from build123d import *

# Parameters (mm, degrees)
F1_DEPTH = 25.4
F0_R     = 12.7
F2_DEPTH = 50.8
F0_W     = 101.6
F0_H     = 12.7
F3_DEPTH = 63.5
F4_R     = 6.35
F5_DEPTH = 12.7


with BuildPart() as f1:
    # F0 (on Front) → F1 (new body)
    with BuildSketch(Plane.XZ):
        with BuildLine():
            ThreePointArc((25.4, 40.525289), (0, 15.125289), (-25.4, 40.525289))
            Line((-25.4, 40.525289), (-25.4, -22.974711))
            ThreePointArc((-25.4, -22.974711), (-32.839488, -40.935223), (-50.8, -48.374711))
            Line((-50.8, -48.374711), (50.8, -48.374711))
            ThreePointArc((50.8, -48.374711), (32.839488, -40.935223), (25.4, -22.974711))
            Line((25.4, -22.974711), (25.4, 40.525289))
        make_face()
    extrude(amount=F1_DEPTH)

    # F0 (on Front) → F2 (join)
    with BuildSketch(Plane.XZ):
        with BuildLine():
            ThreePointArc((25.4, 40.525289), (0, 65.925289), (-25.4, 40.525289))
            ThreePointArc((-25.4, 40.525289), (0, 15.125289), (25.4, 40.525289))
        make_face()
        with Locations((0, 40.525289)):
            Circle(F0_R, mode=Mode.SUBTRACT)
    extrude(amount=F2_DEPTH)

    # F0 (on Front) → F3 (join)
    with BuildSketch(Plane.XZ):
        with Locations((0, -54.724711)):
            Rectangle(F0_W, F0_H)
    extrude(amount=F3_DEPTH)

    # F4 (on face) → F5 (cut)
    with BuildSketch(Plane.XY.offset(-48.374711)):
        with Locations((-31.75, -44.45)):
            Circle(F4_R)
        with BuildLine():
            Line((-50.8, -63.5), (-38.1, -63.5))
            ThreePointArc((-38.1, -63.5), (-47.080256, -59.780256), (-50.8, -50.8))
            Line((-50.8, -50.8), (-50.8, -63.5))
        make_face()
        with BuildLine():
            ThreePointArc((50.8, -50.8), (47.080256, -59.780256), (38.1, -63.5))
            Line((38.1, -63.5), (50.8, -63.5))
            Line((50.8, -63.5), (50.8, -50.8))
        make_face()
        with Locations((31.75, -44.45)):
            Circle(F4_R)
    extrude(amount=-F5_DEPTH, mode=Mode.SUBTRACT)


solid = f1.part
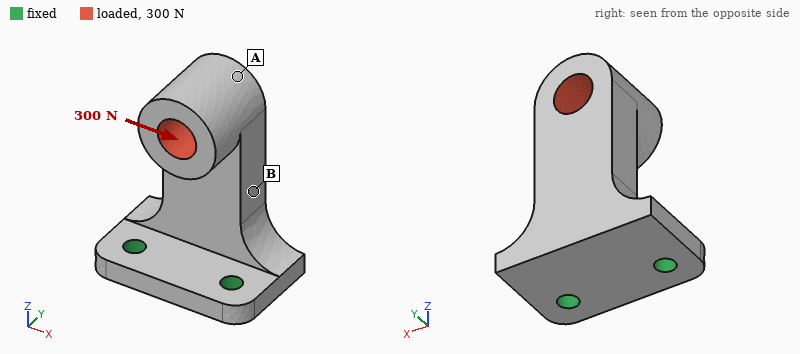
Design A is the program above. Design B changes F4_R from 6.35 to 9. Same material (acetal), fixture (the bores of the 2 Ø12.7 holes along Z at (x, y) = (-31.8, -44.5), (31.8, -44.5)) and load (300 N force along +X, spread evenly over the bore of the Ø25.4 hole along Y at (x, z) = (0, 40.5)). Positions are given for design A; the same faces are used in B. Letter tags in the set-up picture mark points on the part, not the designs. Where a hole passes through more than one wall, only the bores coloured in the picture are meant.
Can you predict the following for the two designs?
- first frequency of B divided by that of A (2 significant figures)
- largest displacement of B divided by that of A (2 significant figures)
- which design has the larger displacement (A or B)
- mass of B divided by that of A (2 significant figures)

1.1
0.88
A
0.99
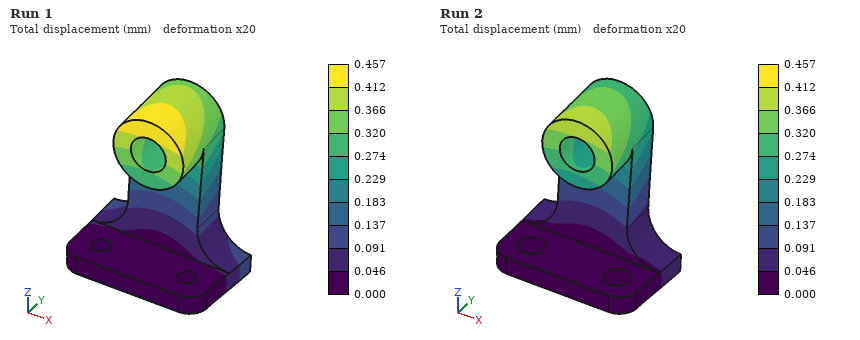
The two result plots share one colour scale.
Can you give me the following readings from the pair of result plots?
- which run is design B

Run 2
